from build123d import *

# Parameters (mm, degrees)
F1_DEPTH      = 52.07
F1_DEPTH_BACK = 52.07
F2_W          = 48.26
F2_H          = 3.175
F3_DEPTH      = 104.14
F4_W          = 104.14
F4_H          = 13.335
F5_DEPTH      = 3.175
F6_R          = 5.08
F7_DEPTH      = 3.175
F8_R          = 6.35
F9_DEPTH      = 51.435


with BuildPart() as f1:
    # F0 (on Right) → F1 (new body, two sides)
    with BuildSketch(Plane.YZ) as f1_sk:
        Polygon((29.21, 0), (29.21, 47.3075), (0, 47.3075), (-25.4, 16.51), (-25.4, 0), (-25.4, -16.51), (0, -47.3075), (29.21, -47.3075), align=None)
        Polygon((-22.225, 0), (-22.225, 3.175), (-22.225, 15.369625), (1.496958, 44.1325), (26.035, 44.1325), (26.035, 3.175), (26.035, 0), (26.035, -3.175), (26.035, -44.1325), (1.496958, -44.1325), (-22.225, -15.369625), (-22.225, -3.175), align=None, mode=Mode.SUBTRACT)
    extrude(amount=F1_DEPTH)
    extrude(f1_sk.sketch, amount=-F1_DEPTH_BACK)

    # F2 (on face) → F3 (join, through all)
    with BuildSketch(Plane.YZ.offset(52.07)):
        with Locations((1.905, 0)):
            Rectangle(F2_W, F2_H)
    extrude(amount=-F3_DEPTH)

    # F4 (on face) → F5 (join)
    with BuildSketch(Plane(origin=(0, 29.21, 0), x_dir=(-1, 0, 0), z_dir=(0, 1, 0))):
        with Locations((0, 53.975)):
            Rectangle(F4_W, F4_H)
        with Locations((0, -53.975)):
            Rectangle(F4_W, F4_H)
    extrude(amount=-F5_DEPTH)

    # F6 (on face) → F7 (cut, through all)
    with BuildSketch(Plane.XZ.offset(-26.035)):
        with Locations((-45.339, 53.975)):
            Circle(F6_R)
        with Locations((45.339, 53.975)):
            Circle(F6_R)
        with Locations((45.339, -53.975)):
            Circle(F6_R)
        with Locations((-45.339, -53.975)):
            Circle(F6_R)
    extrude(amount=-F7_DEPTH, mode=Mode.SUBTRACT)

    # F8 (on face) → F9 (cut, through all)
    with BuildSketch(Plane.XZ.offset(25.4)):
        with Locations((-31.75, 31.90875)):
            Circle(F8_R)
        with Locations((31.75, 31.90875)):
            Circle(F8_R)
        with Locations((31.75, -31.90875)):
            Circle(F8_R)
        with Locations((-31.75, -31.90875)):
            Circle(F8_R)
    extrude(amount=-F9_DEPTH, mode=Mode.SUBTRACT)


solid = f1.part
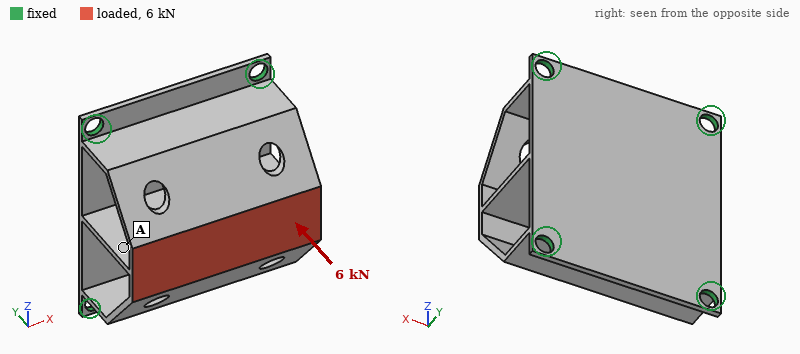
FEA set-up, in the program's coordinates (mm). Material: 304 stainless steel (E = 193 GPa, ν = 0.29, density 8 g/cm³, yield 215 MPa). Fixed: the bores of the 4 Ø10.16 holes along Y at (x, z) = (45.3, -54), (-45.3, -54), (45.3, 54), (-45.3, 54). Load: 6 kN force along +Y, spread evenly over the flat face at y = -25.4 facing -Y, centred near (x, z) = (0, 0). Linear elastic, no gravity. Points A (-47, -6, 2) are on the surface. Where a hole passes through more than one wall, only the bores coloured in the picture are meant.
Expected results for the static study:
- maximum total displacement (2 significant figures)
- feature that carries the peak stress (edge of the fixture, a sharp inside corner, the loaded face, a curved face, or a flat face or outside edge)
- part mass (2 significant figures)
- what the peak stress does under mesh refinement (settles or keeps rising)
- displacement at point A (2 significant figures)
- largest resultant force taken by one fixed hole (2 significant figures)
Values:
0.12 mm
edge of the fixture
850 g
keeps rising
0.11 mm
1.7 kN
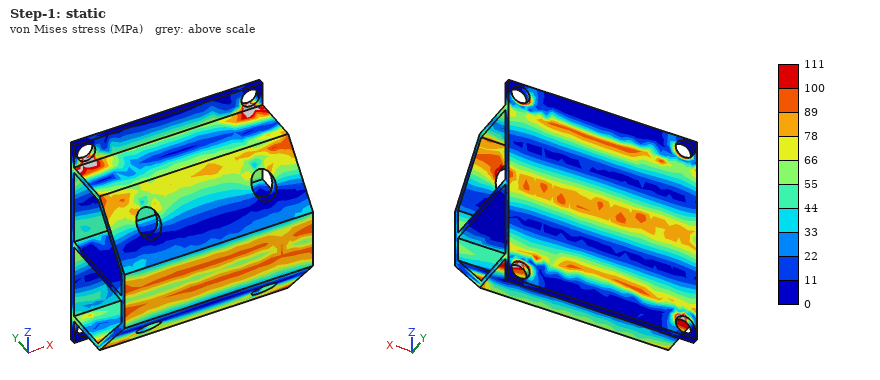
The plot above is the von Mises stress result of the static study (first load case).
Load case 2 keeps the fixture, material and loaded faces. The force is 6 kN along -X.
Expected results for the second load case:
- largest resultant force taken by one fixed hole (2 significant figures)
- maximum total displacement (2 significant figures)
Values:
2.4 kN
82 µm
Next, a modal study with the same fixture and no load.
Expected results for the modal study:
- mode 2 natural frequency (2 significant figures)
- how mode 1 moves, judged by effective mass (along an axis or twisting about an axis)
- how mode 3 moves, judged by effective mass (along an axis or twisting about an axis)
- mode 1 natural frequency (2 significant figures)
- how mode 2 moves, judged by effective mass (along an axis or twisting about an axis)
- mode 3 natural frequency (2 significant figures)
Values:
1800 Hz
along Z
along X
1300 Hz
along Y
2700 Hz
